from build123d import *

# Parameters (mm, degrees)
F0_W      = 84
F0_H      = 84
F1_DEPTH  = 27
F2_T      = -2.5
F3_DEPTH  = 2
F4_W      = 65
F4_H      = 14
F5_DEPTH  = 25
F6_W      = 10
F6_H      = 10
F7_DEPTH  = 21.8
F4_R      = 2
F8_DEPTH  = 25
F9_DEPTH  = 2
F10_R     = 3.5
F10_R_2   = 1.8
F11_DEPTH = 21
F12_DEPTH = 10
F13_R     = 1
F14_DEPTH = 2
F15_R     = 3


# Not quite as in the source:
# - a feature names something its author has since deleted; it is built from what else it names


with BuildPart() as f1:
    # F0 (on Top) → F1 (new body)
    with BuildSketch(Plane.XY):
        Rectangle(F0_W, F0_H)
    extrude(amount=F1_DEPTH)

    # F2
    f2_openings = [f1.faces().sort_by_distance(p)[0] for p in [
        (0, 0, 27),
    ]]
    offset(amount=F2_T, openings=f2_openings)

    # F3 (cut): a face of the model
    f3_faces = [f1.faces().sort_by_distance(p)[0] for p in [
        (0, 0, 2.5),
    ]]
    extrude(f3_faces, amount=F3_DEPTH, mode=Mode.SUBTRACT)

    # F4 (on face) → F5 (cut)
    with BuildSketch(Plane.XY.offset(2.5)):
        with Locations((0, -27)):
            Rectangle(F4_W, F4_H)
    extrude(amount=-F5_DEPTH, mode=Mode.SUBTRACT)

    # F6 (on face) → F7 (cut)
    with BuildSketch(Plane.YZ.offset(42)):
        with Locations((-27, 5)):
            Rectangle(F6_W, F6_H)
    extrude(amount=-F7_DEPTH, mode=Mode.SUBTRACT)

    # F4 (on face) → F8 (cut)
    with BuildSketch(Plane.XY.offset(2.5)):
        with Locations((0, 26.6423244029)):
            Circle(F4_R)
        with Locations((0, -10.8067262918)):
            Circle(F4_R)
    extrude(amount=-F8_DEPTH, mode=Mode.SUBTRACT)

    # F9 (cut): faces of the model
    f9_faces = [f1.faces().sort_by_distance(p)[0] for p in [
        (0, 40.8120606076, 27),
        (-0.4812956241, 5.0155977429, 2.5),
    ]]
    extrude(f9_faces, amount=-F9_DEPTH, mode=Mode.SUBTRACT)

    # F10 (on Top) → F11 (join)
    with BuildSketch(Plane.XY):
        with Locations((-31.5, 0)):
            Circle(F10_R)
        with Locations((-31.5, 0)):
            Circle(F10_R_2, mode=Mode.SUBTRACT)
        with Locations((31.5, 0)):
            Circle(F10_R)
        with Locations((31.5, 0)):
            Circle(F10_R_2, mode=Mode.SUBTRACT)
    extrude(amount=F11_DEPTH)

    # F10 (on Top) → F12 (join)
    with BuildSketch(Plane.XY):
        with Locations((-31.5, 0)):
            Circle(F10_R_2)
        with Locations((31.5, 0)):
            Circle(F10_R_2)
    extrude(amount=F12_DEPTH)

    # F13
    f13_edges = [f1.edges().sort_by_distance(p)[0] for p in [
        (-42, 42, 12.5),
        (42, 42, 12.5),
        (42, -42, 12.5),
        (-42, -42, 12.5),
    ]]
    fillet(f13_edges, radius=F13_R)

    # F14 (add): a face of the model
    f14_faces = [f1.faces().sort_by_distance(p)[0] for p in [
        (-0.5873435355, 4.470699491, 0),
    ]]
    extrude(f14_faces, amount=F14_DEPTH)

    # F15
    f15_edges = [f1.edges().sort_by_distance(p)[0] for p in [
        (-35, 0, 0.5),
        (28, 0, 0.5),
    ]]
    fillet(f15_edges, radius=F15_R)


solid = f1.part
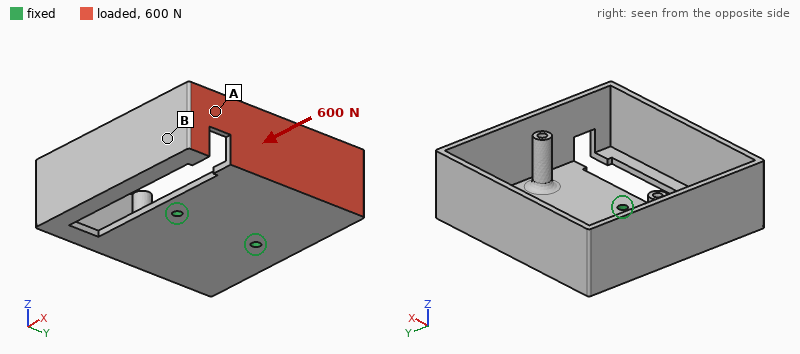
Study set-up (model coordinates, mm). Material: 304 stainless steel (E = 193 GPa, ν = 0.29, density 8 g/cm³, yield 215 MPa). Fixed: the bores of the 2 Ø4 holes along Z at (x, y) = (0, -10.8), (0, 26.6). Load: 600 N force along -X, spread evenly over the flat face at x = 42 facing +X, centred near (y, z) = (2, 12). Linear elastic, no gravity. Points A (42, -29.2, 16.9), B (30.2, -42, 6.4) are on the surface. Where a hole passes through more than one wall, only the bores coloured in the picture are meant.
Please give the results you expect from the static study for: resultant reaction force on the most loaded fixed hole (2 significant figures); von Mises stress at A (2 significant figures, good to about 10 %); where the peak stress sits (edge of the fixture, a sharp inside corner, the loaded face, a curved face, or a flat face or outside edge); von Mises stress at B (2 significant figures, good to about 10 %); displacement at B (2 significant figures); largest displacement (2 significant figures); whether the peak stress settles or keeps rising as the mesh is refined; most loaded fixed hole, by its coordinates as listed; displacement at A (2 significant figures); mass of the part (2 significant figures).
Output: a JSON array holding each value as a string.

["410 N", "39 MPa", "edge of the fixture", "11 MPa", "0.16 mm", "0.25 mm", "keeps rising", "(0, -10.8)", "0.22 mm", "290 g"]
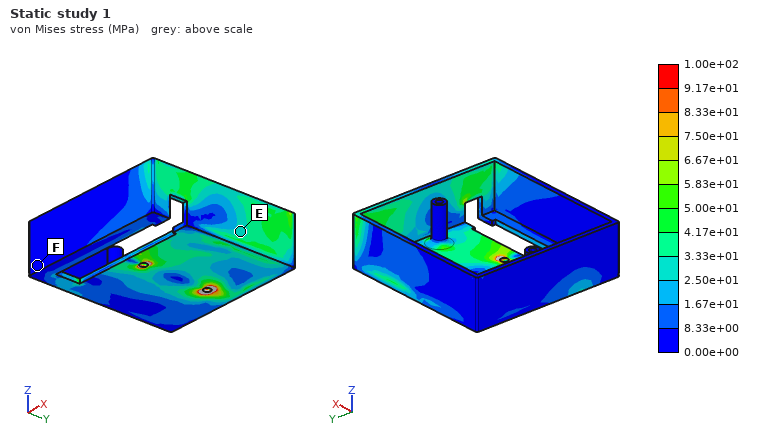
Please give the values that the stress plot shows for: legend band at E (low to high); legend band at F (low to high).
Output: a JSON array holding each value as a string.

["2.50e+01 to 3.33e+01 MPa", "0.00e+00 to 8.33e+00 MPa"]
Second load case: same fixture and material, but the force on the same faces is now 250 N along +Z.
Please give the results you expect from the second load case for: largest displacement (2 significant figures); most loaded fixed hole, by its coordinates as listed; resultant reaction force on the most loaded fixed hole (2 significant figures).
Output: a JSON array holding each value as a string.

["0.35 mm", "(0, -10.8)", "170 N"]
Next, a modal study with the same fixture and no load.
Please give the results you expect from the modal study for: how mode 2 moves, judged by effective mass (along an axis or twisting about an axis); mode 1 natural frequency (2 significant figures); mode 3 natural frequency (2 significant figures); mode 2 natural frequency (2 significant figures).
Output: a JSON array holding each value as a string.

["along Z", "470 Hz", "880 Hz", "500 Hz"]
